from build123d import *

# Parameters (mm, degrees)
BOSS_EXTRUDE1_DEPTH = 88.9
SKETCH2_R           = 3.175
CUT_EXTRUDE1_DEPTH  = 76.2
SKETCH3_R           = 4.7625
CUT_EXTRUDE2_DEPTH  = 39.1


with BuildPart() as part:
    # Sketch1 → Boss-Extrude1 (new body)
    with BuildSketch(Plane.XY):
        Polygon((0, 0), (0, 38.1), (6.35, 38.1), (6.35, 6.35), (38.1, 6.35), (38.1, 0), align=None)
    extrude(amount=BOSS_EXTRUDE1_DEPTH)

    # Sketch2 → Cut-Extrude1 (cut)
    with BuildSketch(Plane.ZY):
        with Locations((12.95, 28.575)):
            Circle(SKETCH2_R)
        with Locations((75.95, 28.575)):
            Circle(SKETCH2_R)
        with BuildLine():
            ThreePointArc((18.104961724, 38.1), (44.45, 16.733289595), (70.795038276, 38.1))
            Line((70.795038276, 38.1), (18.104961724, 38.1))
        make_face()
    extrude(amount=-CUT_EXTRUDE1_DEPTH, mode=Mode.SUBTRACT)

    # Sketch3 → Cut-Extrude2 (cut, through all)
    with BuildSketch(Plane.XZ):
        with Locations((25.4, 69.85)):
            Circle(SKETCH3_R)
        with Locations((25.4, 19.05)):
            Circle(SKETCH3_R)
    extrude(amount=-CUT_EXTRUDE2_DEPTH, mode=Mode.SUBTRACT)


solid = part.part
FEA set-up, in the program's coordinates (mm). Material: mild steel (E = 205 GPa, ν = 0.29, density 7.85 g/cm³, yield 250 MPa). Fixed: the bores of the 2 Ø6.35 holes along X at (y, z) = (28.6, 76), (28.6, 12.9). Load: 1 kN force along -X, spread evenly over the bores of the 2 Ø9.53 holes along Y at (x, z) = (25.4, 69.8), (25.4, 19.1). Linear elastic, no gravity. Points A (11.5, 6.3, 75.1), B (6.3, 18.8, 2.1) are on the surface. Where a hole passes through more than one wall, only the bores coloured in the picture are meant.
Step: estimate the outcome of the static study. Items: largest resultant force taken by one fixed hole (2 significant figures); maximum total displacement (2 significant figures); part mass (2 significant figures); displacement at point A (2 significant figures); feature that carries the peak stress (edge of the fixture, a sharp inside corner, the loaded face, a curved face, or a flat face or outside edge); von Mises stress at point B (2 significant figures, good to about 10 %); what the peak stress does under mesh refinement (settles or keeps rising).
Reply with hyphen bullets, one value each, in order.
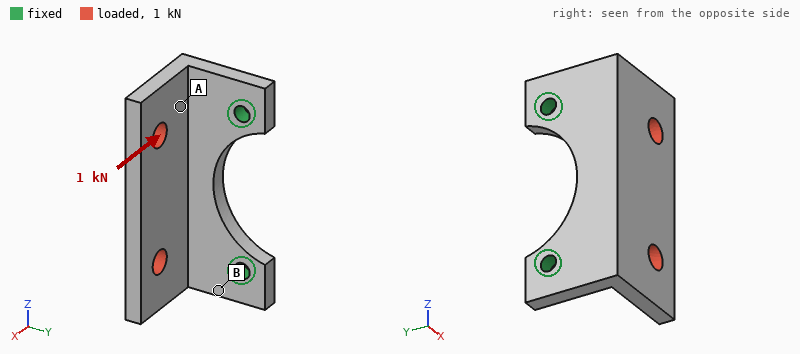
- 500 N
- 53 µm
- 260 g
- 22 µm
- edge of the fixture
- 39 MPa
- keeps rising
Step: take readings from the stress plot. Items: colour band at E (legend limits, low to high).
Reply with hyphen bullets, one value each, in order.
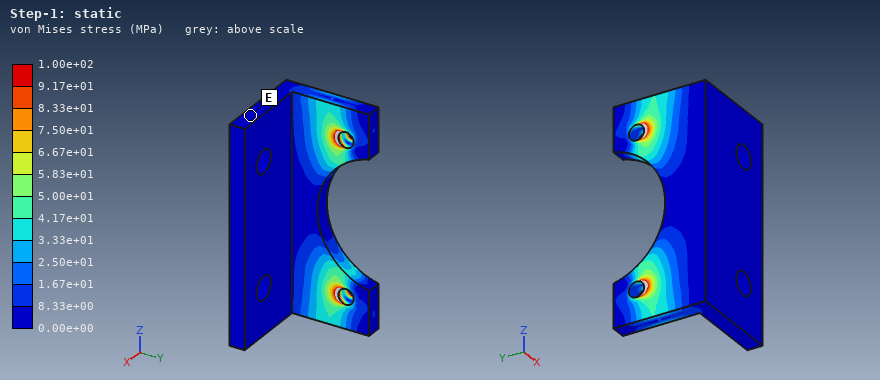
- 0.00e+00 to 8.33e+00 MPa
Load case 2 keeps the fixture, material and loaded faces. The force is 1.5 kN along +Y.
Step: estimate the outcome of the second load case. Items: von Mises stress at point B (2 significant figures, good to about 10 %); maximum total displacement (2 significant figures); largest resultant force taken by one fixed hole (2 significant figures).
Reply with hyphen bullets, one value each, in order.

- 79 MPa
- 0.14 mm
- 800 N
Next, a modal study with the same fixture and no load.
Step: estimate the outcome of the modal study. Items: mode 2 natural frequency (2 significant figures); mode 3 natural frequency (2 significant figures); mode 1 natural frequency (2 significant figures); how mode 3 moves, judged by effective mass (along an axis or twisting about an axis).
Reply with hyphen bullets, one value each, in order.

- 3100 Hz
- 4700 Hz
- 1600 Hz
- along X
